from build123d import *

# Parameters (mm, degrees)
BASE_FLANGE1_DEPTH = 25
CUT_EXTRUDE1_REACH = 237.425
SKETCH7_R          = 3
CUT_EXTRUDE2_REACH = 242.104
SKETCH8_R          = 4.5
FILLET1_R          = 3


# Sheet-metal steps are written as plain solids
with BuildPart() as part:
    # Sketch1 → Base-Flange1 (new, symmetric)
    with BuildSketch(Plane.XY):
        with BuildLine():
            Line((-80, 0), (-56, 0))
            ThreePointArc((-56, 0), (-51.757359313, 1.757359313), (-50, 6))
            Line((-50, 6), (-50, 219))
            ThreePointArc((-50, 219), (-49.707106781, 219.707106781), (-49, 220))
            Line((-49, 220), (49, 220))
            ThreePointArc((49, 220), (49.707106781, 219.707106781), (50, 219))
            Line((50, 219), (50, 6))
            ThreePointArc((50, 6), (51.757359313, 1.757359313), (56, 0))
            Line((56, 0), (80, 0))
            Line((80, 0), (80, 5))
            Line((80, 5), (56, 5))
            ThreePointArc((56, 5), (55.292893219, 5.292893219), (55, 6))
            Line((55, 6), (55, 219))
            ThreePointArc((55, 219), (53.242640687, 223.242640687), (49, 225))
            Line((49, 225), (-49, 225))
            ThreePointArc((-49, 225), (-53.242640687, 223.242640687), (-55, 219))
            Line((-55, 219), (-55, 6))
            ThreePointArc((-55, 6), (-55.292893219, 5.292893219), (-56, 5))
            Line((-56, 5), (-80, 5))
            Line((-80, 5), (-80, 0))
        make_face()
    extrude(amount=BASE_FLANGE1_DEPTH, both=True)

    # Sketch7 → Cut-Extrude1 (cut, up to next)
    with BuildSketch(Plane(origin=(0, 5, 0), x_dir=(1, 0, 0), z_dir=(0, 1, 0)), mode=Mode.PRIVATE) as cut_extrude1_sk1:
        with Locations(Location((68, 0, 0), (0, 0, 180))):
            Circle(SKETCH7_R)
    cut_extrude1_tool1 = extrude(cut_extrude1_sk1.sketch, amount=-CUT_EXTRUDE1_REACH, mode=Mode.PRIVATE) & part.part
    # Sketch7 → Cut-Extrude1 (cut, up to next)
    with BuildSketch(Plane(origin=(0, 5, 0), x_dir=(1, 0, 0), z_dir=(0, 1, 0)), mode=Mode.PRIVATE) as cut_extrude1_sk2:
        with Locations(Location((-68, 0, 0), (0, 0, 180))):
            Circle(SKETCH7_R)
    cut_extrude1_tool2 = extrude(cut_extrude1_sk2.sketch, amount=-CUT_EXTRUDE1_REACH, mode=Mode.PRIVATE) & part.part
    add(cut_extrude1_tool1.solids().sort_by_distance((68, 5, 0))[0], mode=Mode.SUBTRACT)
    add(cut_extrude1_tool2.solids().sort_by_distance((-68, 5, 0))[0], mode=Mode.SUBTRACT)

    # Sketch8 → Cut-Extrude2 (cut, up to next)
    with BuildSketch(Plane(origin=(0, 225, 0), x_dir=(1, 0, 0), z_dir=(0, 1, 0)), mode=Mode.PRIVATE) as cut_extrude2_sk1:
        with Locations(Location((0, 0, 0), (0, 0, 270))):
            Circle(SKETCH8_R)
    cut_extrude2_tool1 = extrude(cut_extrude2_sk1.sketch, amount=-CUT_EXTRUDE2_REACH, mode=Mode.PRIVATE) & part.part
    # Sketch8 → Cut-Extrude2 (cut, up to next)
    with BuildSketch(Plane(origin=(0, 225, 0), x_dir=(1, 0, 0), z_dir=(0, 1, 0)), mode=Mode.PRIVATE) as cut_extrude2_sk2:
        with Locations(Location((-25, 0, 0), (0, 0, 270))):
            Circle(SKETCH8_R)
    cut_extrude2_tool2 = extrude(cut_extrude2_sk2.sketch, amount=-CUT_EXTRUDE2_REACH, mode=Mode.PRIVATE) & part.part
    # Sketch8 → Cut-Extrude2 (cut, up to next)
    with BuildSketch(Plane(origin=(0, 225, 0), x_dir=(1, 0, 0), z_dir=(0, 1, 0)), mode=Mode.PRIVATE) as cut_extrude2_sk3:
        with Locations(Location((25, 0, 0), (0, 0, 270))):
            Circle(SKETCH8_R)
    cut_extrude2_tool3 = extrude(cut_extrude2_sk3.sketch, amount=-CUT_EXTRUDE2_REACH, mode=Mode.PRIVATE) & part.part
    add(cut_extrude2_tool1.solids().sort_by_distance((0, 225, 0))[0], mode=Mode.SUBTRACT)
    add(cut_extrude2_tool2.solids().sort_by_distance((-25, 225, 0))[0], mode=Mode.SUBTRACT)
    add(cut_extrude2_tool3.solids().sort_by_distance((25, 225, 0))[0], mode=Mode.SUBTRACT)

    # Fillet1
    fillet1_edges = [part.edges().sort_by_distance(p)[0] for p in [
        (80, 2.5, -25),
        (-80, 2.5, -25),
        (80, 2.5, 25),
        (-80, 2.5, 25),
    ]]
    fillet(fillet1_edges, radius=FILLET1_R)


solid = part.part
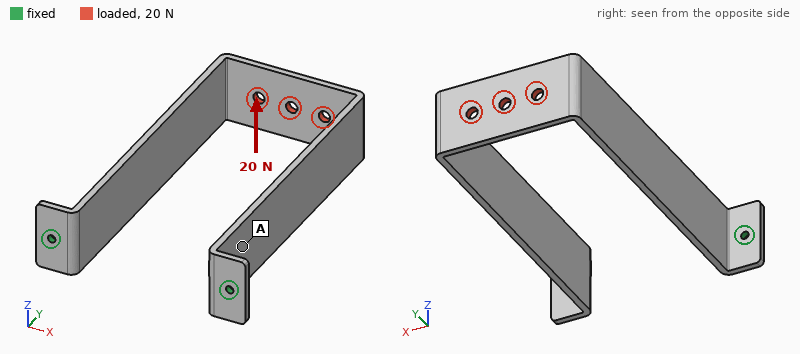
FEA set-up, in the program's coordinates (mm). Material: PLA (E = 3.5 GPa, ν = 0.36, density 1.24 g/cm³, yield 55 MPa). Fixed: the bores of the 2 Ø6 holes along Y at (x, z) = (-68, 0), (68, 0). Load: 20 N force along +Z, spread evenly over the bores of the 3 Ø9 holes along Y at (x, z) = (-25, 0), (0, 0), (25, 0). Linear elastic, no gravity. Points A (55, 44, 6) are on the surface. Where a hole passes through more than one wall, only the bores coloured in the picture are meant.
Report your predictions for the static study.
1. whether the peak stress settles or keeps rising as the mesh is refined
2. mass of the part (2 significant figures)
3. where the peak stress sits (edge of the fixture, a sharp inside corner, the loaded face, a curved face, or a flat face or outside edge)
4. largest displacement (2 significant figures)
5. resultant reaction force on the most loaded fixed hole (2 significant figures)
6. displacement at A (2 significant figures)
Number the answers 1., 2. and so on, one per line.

1. keeps rising
2. 180 g
3. edge of the fixture
4. 3.0 mm
5. 10 N
6. 0.54 mm
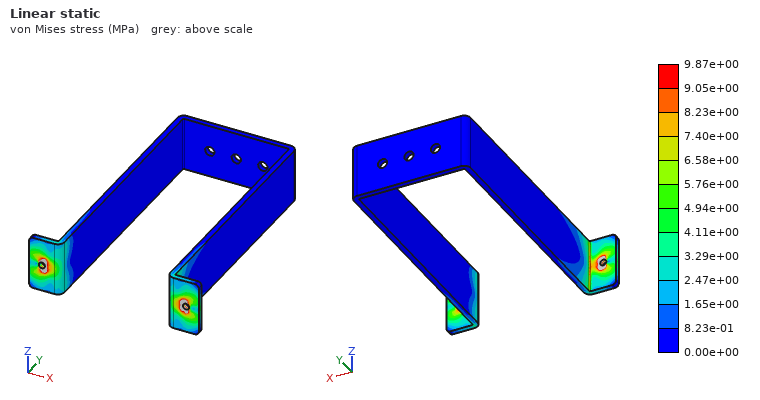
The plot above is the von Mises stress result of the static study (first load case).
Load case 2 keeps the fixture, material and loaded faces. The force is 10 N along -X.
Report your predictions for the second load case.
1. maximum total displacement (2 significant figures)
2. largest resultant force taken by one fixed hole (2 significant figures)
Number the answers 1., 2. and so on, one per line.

1. 3.2 mm
2. 12 N
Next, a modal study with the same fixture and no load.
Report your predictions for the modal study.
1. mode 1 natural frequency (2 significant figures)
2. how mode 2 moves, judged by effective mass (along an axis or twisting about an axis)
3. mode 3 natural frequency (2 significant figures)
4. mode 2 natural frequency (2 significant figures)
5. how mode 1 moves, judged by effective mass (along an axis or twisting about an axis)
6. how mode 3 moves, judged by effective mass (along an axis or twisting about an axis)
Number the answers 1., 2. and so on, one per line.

1. 31 Hz
2. along Z
3. 83 Hz
4. 47 Hz
5. along X
6. twisting about Y
